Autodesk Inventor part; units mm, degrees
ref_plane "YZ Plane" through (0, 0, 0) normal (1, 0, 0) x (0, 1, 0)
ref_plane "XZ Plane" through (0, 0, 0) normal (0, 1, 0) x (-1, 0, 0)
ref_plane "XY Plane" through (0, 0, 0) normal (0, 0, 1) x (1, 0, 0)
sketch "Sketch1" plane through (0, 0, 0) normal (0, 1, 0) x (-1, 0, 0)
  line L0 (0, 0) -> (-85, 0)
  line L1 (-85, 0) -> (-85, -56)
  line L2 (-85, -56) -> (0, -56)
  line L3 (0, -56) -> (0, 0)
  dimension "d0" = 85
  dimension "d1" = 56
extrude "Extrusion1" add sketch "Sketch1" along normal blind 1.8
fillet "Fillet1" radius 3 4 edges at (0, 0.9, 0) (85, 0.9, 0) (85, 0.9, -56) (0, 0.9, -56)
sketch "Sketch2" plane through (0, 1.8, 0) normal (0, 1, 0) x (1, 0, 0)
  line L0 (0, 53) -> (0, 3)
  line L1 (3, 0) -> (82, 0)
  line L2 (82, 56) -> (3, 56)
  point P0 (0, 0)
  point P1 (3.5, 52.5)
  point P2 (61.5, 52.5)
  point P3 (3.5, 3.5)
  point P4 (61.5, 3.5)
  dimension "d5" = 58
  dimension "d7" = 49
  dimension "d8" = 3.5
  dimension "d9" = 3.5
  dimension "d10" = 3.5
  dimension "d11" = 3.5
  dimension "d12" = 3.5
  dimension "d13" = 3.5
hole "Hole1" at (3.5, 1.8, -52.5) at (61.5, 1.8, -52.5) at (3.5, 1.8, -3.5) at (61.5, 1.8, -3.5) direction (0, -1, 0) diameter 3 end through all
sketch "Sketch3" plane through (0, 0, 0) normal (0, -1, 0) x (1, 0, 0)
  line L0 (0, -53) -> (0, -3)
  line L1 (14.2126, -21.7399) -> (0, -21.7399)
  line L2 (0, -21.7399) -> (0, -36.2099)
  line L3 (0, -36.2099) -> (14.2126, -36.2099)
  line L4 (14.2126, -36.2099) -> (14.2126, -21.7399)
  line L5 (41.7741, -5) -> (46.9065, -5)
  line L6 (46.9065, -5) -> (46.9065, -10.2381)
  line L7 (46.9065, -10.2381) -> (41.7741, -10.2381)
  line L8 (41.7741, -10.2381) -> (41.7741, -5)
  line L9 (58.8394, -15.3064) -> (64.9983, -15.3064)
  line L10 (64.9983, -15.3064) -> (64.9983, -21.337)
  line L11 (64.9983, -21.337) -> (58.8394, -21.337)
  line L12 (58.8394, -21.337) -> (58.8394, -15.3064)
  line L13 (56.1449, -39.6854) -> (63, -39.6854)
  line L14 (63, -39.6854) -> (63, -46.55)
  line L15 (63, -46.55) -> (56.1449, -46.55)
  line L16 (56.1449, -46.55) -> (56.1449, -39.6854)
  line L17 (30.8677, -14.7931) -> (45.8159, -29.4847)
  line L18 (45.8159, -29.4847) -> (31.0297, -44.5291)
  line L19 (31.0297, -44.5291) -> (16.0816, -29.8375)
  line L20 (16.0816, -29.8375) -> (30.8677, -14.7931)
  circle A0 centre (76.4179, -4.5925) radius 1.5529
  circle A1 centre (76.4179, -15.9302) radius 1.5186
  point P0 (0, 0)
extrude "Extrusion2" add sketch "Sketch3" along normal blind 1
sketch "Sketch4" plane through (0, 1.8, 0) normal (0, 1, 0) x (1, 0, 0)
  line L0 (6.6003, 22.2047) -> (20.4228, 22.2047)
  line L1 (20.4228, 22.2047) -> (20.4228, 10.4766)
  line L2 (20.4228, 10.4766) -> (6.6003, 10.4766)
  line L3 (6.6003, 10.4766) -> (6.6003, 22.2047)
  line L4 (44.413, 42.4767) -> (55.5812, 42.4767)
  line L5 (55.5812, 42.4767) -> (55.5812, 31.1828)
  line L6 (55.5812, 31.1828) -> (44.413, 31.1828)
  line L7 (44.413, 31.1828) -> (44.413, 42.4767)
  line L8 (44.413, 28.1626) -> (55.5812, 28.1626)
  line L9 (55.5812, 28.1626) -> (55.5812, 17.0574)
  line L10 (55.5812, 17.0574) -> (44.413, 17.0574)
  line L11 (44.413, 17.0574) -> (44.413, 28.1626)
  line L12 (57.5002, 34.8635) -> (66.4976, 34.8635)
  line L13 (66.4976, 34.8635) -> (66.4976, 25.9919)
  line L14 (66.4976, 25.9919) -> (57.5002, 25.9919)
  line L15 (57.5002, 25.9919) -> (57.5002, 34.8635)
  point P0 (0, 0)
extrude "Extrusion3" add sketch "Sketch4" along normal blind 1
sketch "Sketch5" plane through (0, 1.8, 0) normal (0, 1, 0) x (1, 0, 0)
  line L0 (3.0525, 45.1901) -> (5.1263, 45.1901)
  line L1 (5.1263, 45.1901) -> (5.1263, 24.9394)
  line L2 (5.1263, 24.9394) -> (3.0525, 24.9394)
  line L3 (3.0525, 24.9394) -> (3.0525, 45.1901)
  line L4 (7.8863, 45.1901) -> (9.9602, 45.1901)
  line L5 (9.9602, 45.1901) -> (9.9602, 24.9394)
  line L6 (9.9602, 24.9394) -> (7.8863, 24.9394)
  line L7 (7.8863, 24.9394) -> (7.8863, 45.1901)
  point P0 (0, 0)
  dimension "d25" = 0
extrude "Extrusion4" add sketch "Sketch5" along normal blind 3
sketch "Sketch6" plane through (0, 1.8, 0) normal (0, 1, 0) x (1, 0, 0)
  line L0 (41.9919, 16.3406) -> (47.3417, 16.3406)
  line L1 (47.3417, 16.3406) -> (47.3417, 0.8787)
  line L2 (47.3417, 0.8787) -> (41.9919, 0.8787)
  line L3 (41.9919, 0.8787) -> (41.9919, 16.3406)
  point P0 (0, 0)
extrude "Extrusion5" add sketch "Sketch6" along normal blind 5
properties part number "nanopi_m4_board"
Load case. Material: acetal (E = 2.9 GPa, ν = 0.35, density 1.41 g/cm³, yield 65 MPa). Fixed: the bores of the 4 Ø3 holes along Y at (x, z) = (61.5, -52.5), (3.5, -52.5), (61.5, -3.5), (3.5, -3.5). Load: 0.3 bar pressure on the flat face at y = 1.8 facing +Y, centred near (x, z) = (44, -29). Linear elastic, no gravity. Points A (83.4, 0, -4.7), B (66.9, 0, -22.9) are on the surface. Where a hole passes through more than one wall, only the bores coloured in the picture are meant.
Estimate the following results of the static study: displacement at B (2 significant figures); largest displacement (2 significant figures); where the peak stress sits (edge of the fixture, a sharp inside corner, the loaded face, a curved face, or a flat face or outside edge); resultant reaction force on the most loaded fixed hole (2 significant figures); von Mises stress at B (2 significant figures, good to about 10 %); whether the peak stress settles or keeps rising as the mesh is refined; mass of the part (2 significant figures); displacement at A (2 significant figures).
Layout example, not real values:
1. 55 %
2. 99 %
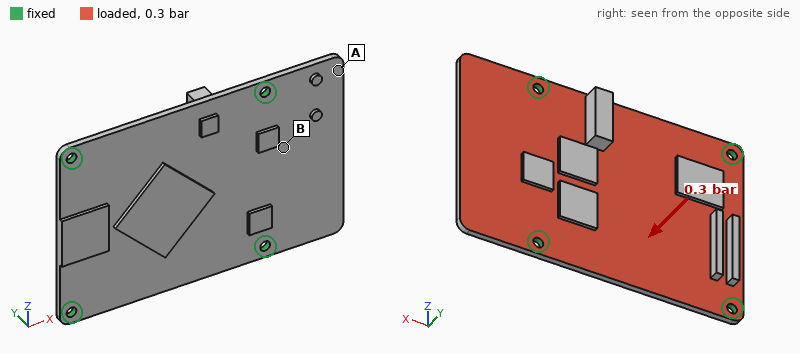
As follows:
1. 0.46 mm
2. 1.1 mm
3. edge of the fixture
4. 41 N
5. 8.4 MPa
6. keeps rising
7. 15 g
8. 0.72 mm
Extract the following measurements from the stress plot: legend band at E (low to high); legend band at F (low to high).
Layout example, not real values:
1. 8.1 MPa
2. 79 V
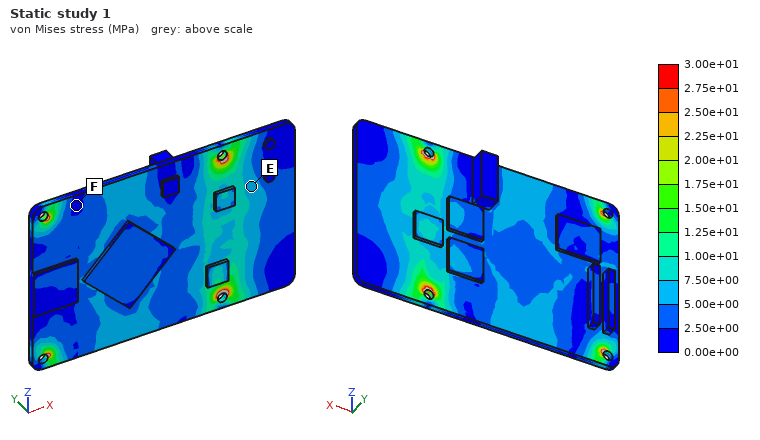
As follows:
1. 5.00e+00 to 7.50e+00 MPa
2. 0.00e+00 to 2.50e+00 MPa
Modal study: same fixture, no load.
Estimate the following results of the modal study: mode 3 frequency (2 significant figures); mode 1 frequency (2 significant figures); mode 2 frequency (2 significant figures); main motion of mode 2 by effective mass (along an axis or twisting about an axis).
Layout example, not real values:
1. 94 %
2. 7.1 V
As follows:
1. 1000 Hz
2. 570 Hz
3. 650 Hz
4. along Y
